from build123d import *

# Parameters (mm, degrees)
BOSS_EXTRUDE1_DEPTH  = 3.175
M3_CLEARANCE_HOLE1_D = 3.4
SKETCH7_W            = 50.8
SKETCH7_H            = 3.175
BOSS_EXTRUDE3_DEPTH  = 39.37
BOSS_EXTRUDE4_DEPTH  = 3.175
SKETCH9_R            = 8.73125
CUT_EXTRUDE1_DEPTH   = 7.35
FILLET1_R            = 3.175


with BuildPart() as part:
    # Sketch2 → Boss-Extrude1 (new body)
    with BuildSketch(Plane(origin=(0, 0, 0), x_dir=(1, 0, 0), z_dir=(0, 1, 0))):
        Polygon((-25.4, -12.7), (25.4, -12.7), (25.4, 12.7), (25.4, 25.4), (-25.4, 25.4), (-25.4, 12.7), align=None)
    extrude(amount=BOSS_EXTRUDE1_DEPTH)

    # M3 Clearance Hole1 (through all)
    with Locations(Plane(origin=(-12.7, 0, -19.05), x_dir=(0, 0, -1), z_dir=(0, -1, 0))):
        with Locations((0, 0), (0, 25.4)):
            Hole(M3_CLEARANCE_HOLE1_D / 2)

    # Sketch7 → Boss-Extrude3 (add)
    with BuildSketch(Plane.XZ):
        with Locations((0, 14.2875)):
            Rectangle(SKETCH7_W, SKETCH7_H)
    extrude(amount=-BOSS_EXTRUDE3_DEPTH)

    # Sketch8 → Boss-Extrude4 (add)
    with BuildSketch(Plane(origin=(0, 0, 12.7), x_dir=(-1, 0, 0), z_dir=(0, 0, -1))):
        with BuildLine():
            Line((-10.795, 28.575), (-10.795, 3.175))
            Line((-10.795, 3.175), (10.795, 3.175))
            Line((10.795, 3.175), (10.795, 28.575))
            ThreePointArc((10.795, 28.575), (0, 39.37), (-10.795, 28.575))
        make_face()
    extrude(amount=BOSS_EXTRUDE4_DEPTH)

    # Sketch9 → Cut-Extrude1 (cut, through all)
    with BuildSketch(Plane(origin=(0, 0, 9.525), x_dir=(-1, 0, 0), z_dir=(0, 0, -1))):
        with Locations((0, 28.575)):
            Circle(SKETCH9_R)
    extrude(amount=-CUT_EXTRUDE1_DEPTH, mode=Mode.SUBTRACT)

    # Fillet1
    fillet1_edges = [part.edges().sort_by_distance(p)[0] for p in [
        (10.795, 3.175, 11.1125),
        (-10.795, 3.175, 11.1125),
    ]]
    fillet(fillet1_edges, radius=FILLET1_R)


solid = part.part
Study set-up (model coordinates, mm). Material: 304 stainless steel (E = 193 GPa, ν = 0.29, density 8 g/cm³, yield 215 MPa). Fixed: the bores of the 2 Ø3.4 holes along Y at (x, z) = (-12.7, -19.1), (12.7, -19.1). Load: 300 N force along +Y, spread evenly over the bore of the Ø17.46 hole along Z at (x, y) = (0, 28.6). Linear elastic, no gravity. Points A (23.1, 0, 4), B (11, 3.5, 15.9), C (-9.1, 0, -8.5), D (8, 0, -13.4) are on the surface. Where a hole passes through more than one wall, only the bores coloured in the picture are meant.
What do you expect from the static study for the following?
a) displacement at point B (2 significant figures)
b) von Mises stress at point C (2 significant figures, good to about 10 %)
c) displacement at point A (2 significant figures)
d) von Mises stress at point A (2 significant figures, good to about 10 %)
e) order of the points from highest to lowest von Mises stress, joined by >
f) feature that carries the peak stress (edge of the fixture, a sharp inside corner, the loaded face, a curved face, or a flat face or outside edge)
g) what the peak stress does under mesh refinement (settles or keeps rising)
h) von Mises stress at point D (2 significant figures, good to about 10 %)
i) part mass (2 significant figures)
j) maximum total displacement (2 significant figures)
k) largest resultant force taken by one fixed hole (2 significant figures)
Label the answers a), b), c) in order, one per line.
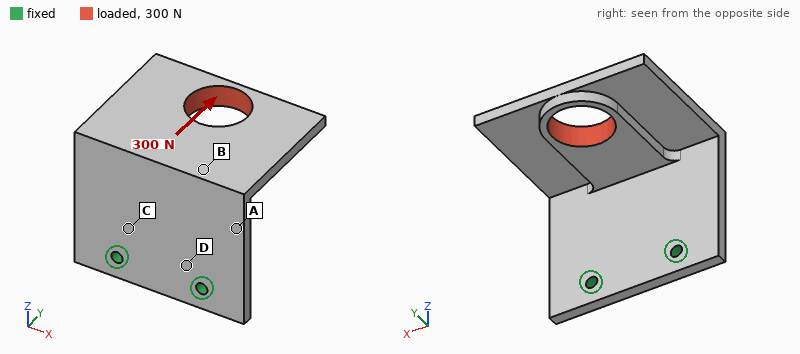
a) 0.15 mm
b) 67 MPa
c) 0.081 mm
d) 32 MPa
e) D > C > A > B
f) edge of the fixture
g) keeps rising
h) 87 MPa
i) 110 g
j) 0.27 mm
k) 150 N
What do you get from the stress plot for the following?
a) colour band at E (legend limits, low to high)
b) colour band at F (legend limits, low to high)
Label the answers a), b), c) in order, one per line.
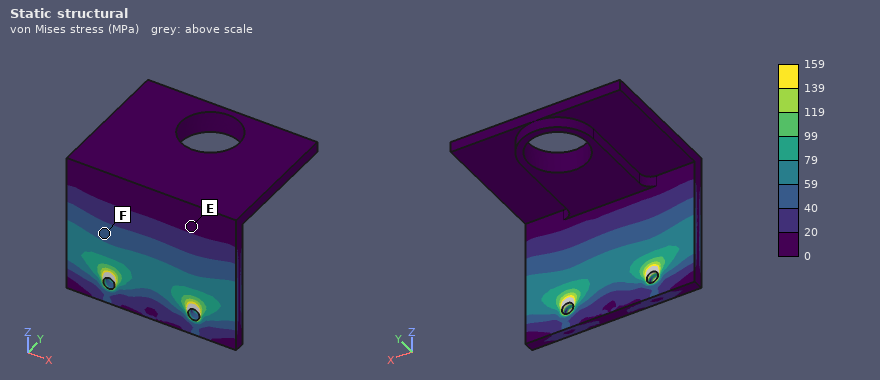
a) 0 to 20 MPa
b) 40 to 59 MPa
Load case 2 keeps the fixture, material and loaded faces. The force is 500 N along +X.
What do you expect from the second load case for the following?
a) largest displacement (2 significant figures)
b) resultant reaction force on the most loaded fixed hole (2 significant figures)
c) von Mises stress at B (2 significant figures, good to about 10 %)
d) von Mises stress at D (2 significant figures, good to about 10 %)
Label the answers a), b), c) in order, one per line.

a) 0.26 mm
b) 750 N
c) 48 MPa
d) 74 MPa
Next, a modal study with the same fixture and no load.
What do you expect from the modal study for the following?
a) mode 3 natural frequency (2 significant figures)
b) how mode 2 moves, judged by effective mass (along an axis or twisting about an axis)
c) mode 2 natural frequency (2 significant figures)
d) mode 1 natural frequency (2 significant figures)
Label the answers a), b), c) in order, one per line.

a) 2300 Hz
b) along X
c) 1300 Hz
d) 670 Hz
